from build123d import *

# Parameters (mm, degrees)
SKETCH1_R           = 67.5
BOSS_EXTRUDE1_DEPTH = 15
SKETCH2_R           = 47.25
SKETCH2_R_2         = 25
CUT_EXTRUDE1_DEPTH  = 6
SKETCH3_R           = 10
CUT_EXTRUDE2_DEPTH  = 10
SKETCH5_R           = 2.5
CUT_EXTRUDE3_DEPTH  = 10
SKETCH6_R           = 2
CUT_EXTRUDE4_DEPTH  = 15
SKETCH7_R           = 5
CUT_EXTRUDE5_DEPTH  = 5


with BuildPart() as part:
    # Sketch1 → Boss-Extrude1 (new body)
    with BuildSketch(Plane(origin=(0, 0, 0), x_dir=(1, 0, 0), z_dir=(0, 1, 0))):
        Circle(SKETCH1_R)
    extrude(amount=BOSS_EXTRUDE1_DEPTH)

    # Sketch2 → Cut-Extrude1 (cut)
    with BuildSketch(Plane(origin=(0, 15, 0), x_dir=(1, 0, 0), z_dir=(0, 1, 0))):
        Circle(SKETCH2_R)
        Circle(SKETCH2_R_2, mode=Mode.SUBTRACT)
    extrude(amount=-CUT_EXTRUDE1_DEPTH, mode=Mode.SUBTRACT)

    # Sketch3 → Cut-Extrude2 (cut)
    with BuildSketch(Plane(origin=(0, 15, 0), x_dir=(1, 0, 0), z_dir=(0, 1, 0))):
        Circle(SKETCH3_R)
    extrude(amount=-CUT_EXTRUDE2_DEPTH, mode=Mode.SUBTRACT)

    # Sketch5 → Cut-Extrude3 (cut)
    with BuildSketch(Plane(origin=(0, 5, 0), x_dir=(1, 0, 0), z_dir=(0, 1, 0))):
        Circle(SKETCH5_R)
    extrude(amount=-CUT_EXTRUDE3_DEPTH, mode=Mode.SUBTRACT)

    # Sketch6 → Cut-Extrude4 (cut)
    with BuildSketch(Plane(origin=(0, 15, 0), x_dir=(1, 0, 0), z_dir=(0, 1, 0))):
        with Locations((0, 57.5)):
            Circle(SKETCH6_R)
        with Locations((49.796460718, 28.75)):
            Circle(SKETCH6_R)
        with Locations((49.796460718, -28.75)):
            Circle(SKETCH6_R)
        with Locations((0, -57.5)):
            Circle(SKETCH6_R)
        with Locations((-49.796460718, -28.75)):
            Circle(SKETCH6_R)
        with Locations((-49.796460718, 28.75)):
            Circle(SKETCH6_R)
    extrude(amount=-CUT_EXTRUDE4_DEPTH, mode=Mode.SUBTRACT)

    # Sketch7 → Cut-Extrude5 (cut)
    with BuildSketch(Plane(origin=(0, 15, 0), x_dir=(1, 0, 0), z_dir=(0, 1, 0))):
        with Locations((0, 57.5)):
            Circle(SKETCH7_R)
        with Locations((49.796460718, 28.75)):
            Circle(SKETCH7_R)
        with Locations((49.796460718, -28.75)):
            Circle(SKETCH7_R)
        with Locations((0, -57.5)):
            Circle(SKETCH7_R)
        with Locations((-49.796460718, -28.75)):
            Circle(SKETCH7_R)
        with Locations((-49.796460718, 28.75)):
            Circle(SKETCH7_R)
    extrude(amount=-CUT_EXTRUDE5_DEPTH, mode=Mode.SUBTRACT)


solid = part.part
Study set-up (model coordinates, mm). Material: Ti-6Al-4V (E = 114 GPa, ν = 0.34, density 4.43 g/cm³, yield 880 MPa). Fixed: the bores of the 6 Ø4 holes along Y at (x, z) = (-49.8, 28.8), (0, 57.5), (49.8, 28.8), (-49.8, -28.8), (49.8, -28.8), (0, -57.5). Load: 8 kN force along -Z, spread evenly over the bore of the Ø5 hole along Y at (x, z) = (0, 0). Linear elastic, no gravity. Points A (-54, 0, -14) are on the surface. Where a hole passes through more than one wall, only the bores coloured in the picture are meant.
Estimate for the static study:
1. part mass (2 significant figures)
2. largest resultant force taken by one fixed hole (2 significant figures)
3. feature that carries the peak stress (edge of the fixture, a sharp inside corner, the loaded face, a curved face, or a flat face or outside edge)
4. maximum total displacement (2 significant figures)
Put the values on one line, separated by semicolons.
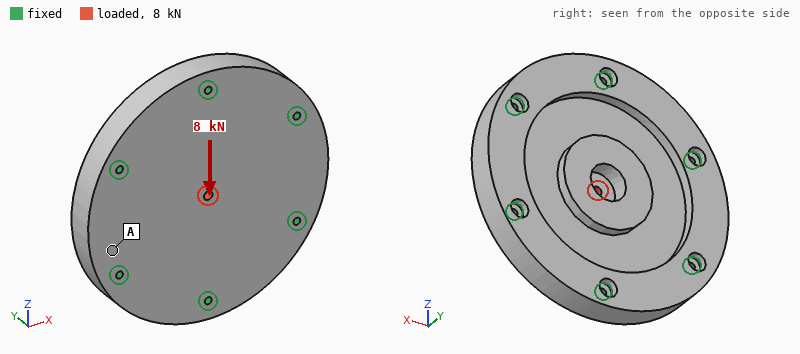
790 g; 1.9 kN; the loaded face; 10 µm
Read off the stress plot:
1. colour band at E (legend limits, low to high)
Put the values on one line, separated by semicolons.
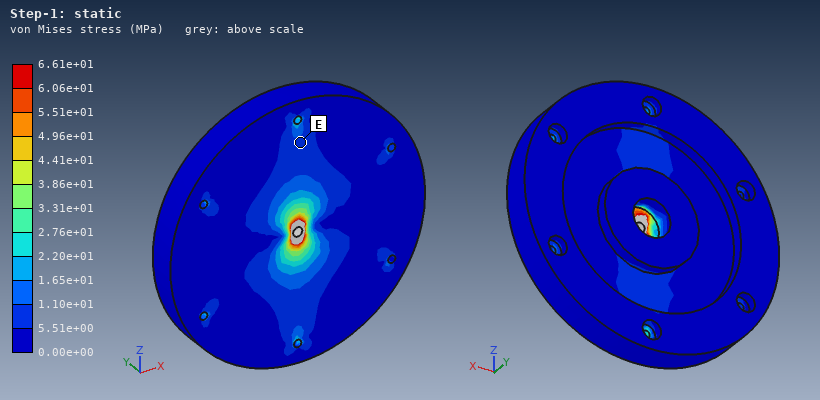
5.51e+00 to 1.10e+01 MPa
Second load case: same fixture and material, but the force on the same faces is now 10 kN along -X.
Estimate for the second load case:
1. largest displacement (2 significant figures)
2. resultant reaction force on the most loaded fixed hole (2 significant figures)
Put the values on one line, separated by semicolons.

13 µm; 2.1 kN
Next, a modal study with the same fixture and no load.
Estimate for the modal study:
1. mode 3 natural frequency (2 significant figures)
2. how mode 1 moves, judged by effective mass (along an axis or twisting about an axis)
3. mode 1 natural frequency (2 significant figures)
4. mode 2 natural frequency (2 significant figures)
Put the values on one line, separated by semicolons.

10 kHz; along Y; 5800 Hz; 10 kHz
